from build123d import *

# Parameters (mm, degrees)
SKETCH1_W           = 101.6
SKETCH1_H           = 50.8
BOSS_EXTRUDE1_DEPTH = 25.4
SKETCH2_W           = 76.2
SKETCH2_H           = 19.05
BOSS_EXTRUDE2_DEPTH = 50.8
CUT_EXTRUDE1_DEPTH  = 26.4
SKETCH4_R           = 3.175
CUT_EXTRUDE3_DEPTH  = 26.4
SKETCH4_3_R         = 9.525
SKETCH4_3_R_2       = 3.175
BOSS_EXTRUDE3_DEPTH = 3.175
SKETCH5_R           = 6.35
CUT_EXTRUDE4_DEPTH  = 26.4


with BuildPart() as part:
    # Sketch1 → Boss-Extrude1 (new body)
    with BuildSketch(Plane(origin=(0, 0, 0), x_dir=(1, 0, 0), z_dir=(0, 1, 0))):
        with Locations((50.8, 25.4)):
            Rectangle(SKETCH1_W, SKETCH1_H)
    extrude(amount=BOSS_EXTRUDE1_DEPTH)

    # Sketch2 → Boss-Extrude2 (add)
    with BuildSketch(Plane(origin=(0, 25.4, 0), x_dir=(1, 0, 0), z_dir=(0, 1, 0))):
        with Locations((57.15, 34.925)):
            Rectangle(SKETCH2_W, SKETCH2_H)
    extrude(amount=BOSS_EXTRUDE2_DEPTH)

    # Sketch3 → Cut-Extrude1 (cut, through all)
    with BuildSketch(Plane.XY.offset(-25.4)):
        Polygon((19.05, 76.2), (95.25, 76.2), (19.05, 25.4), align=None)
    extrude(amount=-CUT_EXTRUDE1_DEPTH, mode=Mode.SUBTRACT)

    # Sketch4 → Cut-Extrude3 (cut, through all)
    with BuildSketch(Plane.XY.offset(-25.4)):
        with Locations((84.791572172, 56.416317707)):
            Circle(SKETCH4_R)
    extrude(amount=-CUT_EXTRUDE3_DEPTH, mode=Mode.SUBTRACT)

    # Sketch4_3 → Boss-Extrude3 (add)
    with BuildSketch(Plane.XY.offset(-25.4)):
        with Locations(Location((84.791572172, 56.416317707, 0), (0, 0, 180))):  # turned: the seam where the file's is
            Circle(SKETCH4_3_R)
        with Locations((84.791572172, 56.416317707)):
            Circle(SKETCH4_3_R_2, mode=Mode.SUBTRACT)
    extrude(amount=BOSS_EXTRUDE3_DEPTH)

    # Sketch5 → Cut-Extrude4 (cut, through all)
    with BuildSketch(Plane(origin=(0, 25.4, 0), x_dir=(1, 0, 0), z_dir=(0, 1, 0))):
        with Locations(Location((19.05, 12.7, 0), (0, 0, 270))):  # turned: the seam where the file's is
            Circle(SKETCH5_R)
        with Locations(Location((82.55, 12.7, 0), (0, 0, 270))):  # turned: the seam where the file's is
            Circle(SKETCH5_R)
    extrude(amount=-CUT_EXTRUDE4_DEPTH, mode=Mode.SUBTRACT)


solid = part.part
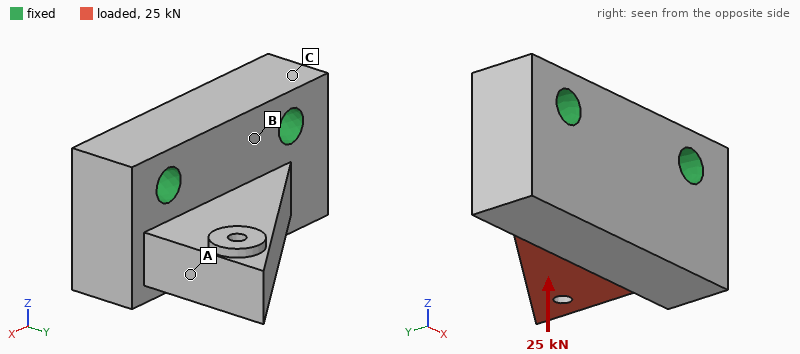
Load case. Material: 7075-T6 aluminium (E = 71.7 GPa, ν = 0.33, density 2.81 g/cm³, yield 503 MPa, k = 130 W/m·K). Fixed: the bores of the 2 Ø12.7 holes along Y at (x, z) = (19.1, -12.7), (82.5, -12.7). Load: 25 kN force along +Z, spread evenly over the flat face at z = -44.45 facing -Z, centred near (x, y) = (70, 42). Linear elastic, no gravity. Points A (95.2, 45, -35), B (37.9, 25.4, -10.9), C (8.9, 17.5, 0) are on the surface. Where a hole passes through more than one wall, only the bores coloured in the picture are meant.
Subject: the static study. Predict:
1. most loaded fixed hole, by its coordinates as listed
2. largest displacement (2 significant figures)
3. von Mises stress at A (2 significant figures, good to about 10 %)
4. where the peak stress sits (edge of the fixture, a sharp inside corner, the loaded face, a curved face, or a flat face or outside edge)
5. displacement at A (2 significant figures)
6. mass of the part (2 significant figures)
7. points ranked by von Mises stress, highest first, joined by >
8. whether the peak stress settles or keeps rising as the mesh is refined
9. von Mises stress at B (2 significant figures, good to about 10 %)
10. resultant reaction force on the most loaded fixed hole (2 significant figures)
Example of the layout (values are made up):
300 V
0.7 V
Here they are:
(82.5, -12.7)
0.36 mm
54 MPa
edge of the fixture
0.14 mm
450 g
A > B > C
keeps rising
36 MPa
20 kN
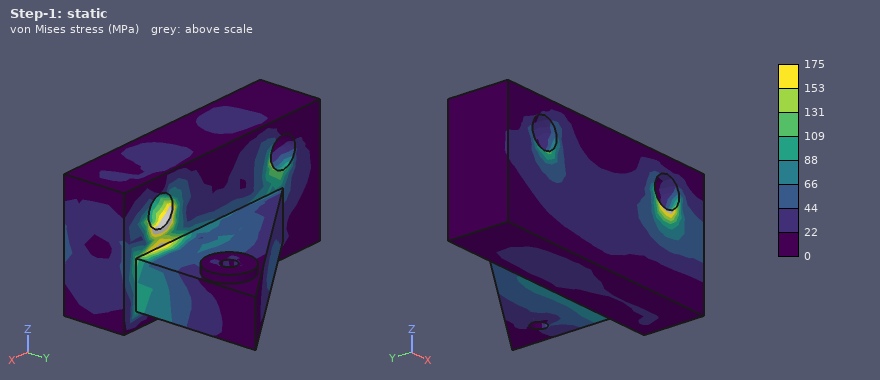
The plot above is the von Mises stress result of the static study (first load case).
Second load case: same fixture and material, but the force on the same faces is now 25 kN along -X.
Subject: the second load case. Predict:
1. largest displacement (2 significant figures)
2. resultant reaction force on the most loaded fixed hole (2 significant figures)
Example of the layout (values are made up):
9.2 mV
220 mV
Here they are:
0.11 mm
20 kN
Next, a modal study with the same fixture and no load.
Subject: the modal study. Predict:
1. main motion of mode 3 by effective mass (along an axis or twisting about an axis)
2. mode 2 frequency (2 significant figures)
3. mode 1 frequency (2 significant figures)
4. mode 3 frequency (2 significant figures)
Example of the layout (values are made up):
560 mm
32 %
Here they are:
along Y
9500 Hz
5400 Hz
10 kHz
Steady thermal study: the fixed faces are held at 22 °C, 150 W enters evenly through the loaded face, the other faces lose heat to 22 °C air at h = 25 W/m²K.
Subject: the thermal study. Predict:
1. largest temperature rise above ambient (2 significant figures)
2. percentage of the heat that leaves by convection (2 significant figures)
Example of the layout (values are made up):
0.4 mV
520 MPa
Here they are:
45 K
4.0 %
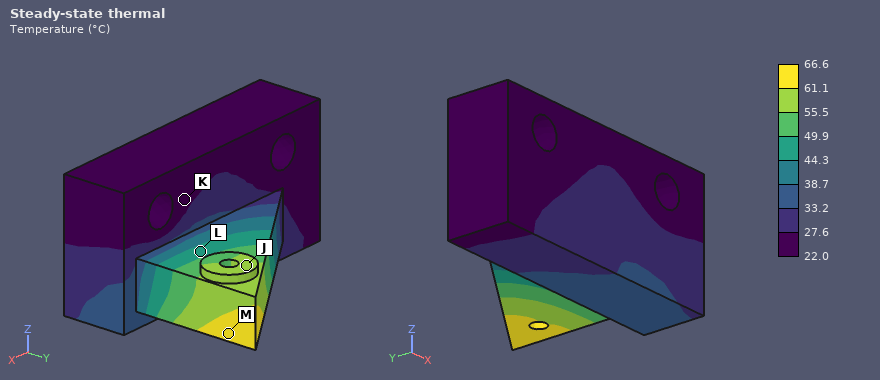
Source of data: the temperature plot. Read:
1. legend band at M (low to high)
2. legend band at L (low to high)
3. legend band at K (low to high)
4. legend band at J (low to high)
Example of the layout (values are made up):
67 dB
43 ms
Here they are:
61.1 to 66.6 °C
44.3 to 49.9 °C
22.0 to 27.6 °C
55.5 to 61.1 °C
